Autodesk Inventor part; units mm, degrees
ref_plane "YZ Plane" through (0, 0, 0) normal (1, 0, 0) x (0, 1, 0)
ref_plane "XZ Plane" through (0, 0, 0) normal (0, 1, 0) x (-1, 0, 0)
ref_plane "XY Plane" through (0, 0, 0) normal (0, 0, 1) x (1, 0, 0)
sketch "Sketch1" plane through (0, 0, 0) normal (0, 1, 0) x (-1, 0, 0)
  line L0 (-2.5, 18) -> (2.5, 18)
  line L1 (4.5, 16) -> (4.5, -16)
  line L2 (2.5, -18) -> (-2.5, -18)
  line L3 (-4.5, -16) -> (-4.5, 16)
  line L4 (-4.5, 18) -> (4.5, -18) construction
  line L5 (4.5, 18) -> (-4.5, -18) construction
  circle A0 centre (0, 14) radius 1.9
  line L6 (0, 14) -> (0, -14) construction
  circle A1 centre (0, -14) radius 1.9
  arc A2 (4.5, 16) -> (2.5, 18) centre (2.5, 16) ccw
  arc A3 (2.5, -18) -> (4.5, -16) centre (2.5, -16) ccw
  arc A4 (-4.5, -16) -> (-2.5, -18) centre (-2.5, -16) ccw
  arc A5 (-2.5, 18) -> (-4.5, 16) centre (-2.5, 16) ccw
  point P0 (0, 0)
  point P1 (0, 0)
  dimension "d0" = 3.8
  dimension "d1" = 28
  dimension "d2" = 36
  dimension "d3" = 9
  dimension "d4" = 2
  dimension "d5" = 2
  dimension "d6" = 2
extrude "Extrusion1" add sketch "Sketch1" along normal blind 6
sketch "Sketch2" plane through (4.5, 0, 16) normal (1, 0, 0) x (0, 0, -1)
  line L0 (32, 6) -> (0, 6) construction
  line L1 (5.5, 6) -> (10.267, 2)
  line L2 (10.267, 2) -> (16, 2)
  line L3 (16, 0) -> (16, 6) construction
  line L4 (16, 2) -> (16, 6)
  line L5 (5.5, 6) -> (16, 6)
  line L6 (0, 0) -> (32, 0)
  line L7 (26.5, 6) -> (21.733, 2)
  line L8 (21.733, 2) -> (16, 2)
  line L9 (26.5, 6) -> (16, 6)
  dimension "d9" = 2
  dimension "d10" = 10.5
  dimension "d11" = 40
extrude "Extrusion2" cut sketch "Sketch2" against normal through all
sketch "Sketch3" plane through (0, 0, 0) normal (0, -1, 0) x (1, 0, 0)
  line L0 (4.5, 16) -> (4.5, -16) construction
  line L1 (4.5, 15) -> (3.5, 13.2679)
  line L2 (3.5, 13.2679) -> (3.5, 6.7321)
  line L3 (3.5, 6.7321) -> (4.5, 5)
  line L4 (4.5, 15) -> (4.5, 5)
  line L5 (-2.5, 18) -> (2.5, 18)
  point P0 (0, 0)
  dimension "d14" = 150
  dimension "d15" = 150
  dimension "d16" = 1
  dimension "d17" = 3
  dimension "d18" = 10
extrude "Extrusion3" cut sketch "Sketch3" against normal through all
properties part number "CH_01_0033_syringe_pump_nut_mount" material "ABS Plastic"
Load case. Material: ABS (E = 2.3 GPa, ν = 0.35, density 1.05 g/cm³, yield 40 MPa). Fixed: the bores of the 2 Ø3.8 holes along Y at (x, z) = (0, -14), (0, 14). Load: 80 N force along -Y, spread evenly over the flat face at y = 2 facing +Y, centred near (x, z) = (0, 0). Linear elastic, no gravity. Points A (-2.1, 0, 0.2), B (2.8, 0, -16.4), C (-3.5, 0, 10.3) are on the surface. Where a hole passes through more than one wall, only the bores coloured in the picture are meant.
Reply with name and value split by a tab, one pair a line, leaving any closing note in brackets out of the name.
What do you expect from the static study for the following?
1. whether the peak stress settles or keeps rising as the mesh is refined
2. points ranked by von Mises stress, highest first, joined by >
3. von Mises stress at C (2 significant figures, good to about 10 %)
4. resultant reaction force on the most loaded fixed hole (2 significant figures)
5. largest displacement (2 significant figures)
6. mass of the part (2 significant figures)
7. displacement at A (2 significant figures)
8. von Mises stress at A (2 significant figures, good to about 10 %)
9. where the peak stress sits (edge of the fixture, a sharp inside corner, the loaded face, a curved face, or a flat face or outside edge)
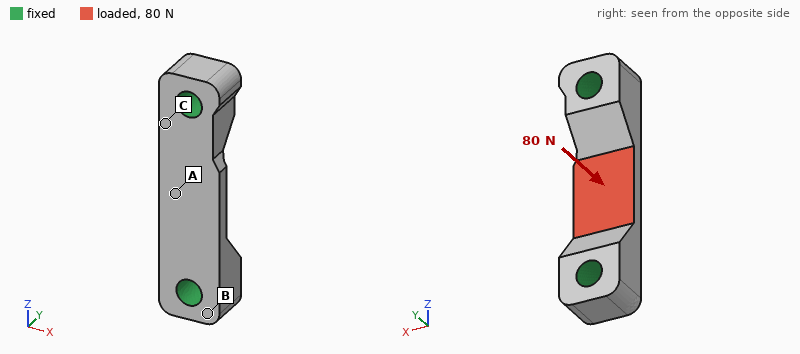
whether the peak stress settles or keeps rising as the mesh is refined	keeps rising
points ranked by von Mises stress, highest first, joined by >	A > C > B
von Mises stress at C	3.6 MPa
resultant reaction force on the most loaded fixed hole	53 N
largest displacement	0.10 mm
mass of the part	1.2 g
displacement at A	0.091 mm
von Mises stress at A	12 MPa
where the peak stress sits	a sharp inside corner
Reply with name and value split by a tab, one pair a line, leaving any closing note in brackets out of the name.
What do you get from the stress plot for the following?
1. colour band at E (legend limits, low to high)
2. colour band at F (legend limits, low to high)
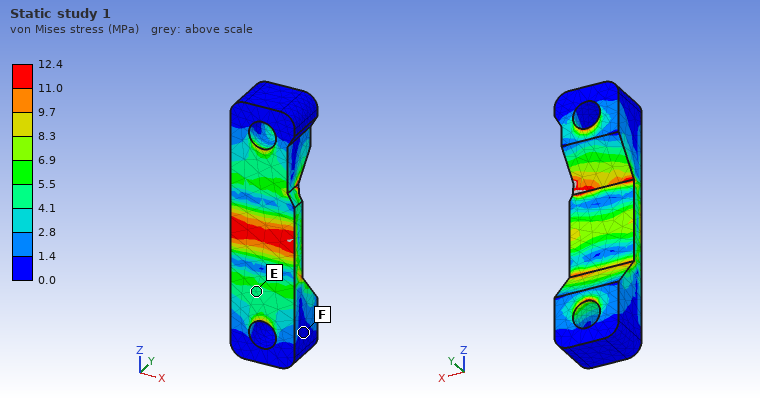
colour band at E	4.1 to 5.5 MPa
colour band at F	0.0 to 1.4 MPa
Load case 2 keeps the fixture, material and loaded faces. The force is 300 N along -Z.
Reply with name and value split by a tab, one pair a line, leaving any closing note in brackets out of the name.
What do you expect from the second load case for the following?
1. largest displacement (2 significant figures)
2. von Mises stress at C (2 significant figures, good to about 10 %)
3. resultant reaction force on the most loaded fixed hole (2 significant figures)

largest displacement	54 µm
von Mises stress at C	7.4 MPa
resultant reaction force on the most loaded fixed hole	160 N
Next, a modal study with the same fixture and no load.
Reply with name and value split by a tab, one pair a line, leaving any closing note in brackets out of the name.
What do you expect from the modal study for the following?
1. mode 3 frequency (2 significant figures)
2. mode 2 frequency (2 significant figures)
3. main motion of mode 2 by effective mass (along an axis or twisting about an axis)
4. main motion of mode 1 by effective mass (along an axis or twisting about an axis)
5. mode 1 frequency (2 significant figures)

mode 3 frequency	15 kHz
mode 2 frequency	13 kHz
main motion of mode 2 by effective mass	along X
main motion of mode 1 by effective mass	along Y
mode 1 frequency	11 kHz
